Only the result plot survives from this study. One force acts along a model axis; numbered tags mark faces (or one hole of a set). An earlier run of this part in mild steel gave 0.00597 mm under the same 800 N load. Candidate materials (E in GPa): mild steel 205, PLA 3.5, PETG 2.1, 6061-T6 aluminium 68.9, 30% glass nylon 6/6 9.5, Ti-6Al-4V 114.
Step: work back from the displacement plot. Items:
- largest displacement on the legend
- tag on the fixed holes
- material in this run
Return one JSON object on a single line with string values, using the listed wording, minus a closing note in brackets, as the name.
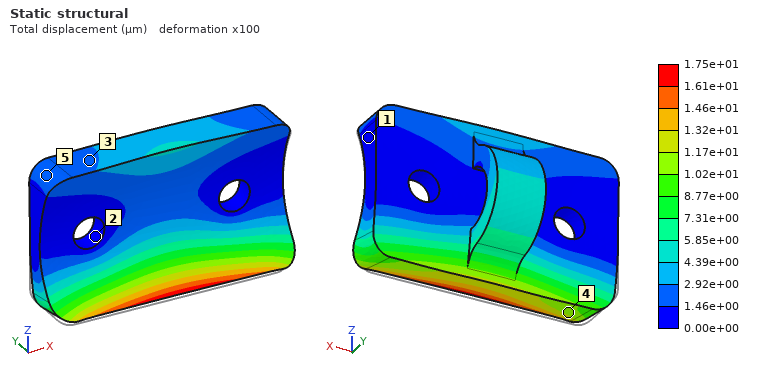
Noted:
{"largest displacement on the legend": "1.75e+01 µm", "tag on the fixed holes": "2", "material in this run": "6061-T6 aluminium"}
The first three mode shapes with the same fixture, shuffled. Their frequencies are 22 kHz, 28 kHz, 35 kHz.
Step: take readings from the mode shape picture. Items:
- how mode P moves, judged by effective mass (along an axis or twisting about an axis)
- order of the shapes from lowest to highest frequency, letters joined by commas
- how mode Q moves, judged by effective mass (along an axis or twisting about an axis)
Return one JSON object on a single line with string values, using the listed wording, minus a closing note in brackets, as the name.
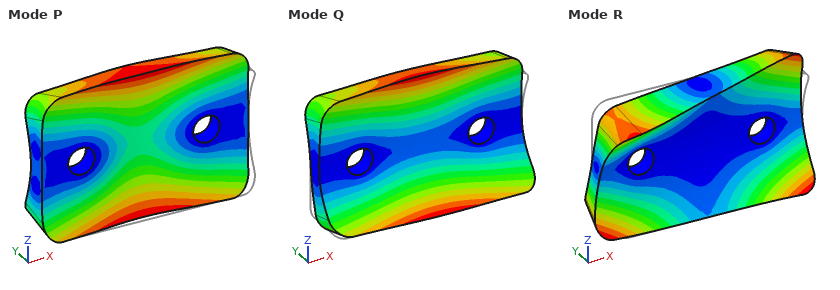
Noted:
{"how mode P moves, judged by effective mass": "along Y", "order of the shapes from lowest to highest frequency, letters joined by commas": "Q, P, R", "how mode Q moves, judged by effective mass": "twisting about X"}
